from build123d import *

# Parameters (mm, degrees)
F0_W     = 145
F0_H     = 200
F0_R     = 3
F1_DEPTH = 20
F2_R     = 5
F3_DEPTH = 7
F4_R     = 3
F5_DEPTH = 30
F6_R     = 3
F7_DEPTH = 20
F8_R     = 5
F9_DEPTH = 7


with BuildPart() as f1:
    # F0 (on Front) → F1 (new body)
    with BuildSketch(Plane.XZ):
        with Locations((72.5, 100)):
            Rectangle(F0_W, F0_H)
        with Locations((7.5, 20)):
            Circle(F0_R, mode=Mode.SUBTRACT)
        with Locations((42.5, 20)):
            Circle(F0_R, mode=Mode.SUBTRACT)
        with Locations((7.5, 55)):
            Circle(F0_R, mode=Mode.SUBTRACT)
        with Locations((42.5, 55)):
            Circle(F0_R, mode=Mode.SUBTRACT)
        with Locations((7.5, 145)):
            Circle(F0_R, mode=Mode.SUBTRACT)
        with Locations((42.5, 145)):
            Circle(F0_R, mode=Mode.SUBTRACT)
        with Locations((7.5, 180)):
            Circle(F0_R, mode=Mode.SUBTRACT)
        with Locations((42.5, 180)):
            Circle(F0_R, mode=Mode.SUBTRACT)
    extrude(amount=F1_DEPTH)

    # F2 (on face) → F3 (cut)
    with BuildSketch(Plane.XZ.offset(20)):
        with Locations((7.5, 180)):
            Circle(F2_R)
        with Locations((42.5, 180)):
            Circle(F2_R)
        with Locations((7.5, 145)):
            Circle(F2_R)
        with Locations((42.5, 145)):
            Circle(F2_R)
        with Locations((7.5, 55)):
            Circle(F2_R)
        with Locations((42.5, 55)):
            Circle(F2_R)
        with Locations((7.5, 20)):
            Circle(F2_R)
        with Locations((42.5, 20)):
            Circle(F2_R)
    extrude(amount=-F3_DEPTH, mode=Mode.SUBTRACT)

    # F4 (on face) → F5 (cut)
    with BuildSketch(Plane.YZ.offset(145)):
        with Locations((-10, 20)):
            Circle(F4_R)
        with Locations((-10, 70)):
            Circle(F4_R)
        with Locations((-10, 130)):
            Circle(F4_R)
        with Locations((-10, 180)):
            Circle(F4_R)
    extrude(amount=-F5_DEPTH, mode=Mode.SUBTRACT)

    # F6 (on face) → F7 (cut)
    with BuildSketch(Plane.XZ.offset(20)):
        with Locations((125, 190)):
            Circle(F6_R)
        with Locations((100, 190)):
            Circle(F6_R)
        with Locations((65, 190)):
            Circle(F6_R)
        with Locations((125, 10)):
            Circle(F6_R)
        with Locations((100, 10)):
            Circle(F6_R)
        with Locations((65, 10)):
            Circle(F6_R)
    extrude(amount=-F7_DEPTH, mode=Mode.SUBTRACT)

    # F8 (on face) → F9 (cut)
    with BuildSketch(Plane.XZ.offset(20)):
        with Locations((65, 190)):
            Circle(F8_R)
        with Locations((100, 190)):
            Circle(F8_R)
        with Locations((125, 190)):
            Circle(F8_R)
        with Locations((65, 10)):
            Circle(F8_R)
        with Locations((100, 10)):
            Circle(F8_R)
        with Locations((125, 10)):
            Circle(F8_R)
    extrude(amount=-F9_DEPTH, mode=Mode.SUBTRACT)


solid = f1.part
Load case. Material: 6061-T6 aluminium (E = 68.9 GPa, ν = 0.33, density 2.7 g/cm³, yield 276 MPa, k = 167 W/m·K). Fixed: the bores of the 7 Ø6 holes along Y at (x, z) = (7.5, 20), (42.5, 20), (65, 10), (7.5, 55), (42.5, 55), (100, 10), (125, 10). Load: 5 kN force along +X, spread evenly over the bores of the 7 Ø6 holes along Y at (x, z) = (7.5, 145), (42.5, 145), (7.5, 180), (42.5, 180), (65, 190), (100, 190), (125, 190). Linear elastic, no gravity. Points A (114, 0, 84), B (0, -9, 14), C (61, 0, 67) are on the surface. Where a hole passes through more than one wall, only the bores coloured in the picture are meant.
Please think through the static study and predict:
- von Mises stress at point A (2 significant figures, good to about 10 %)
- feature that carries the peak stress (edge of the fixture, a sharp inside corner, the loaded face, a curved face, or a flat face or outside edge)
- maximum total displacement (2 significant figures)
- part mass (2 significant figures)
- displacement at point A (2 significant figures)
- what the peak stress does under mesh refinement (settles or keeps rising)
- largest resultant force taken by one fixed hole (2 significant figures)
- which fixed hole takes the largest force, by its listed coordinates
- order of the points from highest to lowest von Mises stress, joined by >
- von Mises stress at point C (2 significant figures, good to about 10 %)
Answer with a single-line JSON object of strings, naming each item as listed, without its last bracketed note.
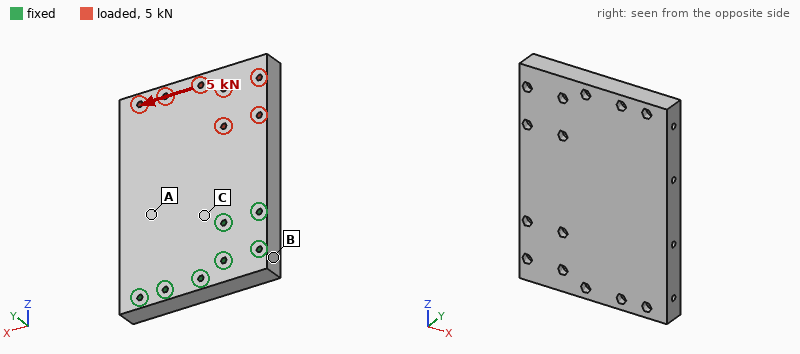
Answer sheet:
{"von Mises stress at point A": "5.0 MPa", "feature that carries the peak stress": "edge of the fixture", "maximum total displacement": "45 µm", "part mass": "1.5 kg", "displacement at point A": "12 µm", "what the peak stress does under mesh refinement": "keeps rising", "largest resultant force taken by one fixed hole": "4.4 kN", "which fixed hole takes the largest force, by its listed coordinates": "(7.5, 55)", "order of the points from highest to lowest von Mises stress, joined by >": "C > A > B", "von Mises stress at point C": "7.2 MPa"}
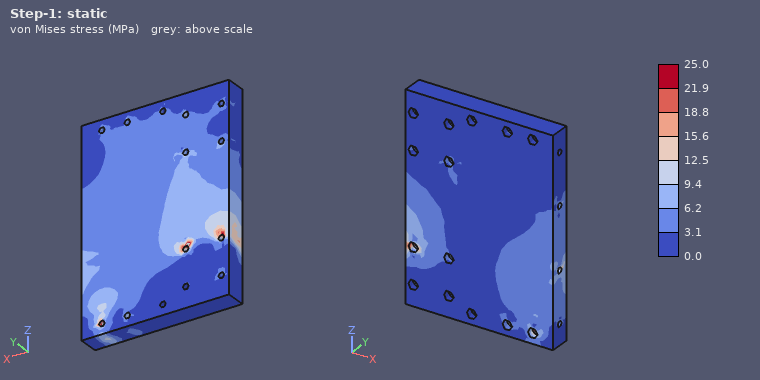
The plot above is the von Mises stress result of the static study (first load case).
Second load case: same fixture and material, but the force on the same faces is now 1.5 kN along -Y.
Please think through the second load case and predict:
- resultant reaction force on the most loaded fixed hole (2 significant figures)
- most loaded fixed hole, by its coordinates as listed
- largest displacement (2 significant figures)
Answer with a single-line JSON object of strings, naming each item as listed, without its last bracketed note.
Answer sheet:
{"resultant reaction force on the most loaded fixed hole": "4.1 kN", "most loaded fixed hole, by its coordinates as listed": "(42.5, 55)", "largest displacement": "0.26 mm"}
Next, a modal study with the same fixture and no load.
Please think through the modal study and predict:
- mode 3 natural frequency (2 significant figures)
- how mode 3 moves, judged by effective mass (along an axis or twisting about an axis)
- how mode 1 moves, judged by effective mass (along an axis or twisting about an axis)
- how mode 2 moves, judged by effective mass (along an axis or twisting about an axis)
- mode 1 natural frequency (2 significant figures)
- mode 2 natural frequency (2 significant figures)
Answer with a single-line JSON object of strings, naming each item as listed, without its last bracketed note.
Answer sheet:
{"mode 3 natural frequency": "2800 Hz", "how mode 3 moves, judged by effective mass": "along X", "how mode 1 moves, judged by effective mass": "along Y", "how mode 2 moves, judged by effective mass": "twisting about Z", "mode 1 natural frequency": "590 Hz", "mode 2 natural frequency": "1400 Hz"}
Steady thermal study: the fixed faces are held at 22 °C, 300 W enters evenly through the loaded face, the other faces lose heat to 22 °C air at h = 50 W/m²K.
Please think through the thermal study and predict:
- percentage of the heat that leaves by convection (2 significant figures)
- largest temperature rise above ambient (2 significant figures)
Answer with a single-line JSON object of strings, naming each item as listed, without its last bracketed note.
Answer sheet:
{"percentage of the heat that leaves by convection": "37 %", "largest temperature rise above ambient": "71 K"}
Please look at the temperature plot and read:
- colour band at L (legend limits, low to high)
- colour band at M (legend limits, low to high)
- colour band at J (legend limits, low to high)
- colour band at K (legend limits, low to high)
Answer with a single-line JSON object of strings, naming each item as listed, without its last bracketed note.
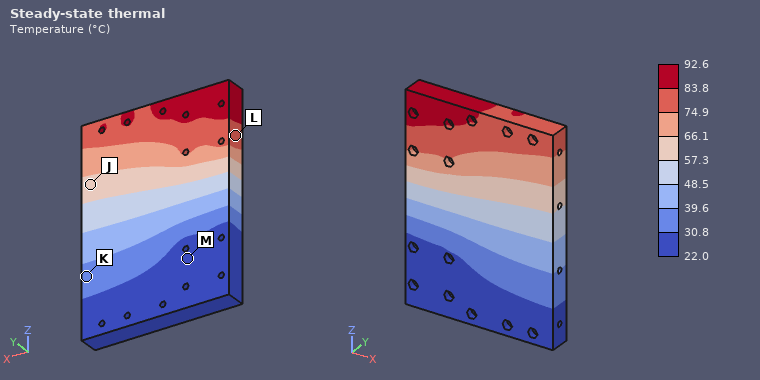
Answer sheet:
{"colour band at L": "74.9 to 83.8 °C", "colour band at M": "22.0 to 30.8 °C", "colour band at J": "57.3 to 66.1 °C", "colour band at K": "30.8 to 39.6 °C"}
